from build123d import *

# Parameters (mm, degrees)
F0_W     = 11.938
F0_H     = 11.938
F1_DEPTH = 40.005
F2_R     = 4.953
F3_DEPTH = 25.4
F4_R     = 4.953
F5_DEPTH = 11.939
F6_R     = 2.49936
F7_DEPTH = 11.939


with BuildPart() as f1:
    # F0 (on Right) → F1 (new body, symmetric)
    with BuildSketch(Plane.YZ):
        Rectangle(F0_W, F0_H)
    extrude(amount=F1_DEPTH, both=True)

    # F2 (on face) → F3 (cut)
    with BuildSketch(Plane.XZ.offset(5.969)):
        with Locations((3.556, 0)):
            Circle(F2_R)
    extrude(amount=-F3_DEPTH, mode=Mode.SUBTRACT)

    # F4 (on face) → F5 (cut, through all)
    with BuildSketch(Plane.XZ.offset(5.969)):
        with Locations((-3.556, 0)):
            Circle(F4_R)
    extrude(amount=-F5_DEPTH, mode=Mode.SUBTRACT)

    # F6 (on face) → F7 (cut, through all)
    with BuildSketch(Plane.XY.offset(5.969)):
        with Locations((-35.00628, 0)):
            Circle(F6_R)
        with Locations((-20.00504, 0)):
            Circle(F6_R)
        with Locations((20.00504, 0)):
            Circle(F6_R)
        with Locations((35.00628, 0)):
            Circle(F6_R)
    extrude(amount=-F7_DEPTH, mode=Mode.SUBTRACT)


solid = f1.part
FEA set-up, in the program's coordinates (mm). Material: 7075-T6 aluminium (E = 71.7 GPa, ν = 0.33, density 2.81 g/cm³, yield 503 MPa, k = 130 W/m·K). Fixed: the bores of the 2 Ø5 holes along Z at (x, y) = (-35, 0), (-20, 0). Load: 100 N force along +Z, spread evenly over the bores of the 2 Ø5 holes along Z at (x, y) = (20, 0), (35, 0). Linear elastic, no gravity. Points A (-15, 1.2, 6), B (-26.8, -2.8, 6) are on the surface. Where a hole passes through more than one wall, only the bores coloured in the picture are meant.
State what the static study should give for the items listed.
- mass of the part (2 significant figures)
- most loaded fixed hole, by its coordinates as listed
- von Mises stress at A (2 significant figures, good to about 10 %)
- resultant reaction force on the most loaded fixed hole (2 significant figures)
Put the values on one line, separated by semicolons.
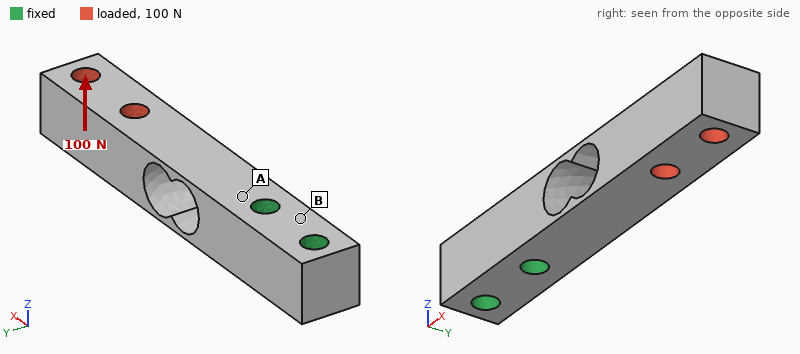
25 g; (-20, 0); 18 MPa; 120 N
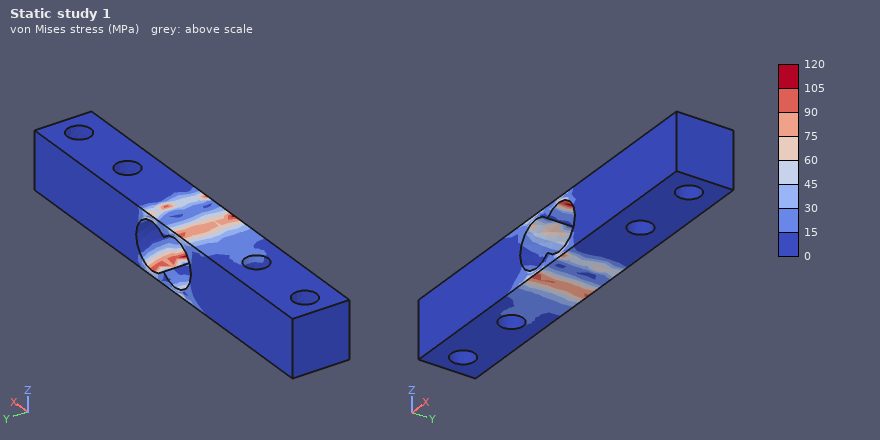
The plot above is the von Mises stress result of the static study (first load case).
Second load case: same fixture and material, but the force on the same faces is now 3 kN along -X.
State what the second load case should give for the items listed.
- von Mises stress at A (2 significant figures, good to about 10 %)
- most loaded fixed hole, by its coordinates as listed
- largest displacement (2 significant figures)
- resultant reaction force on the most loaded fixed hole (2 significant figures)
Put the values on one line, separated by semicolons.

36 MPa; (-20, 0); 41 µm; 2.8 kN
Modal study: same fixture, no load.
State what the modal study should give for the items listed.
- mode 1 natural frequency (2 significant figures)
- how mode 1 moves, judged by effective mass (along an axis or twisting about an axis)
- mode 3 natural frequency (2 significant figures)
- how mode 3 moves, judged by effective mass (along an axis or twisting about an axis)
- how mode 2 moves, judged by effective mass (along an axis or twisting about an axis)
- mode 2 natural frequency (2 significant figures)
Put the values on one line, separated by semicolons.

1400 Hz; along Z; 6700 Hz; twisting about X; along Y; 1700 Hz
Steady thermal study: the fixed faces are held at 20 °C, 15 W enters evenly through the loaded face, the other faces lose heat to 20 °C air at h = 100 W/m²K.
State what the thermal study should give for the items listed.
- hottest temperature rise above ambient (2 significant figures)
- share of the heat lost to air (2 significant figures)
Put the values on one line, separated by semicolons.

45 K; 55 %
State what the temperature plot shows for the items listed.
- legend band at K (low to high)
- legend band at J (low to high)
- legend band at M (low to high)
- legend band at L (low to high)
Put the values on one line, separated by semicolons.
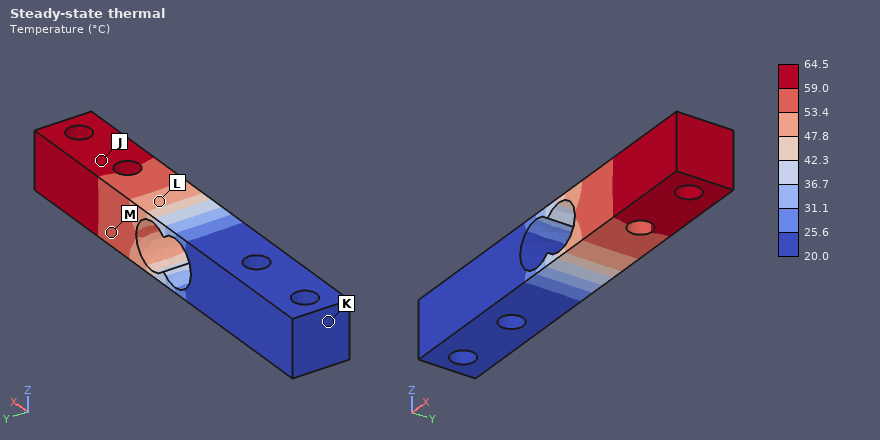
20.0 to 25.6 °C; 59.0 to 64.5 °C; 53.4 to 59.0 °C; 47.8 to 53.4 °C
